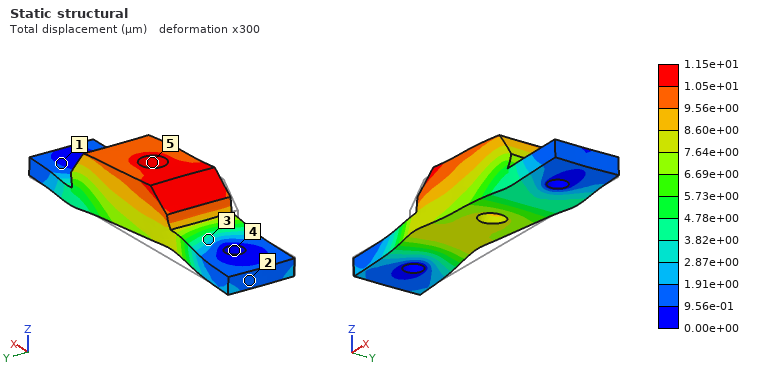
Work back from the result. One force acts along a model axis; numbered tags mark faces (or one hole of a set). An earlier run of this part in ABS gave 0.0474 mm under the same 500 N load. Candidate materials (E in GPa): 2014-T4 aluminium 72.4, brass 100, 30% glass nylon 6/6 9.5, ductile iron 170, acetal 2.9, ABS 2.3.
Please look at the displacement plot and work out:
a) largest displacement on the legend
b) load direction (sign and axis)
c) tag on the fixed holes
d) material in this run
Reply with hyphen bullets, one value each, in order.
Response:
- 1.15e+01 µm
- +X
- 4
- 30% glass nylon 6/6
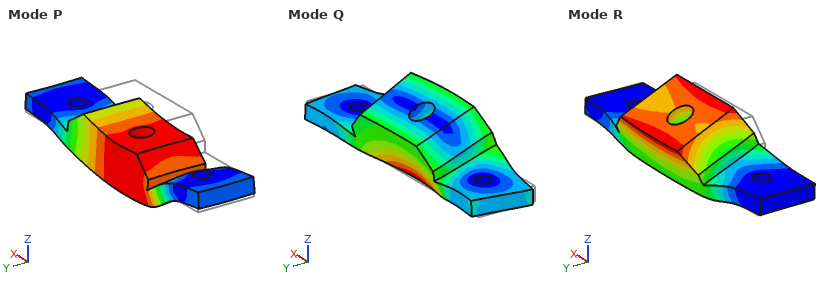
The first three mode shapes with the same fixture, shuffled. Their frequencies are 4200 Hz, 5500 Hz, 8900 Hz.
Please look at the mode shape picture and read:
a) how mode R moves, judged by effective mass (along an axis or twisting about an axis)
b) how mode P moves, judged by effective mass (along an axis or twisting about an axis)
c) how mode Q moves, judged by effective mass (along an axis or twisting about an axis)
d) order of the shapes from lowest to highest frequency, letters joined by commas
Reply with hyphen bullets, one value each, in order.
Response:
- along Y
- along Z
- along Y
- R, P, Q
